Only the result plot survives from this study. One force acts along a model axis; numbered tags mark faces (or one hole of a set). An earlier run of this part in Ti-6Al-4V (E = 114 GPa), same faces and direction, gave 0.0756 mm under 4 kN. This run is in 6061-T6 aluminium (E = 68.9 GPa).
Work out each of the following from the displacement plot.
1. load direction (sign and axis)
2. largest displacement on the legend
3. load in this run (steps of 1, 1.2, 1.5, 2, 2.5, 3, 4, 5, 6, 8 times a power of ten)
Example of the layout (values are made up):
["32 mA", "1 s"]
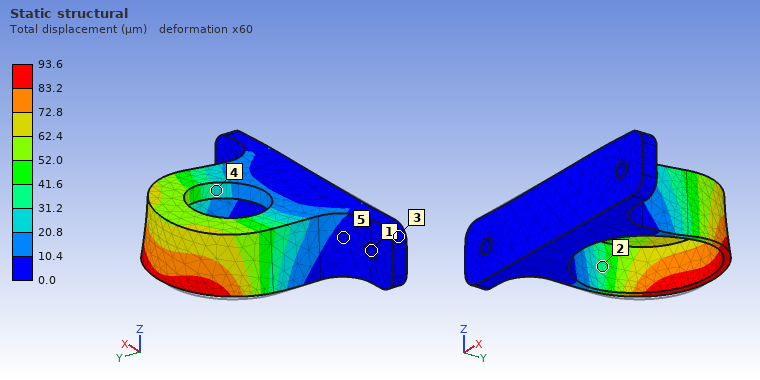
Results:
["+X", "93.6 µm", "3 kN"]
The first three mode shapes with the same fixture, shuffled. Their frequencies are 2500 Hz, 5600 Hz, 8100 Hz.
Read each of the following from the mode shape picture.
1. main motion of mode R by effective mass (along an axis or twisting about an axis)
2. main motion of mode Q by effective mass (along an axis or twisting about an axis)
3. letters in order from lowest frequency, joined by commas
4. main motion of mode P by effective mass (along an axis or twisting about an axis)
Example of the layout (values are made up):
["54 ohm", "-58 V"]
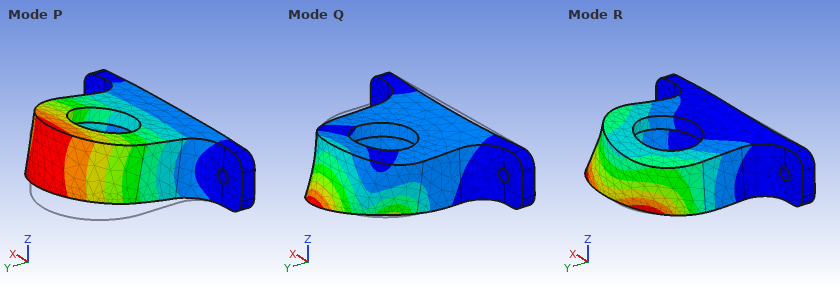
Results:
["along X", "along Y", "P, R, Q", "along Z"]
